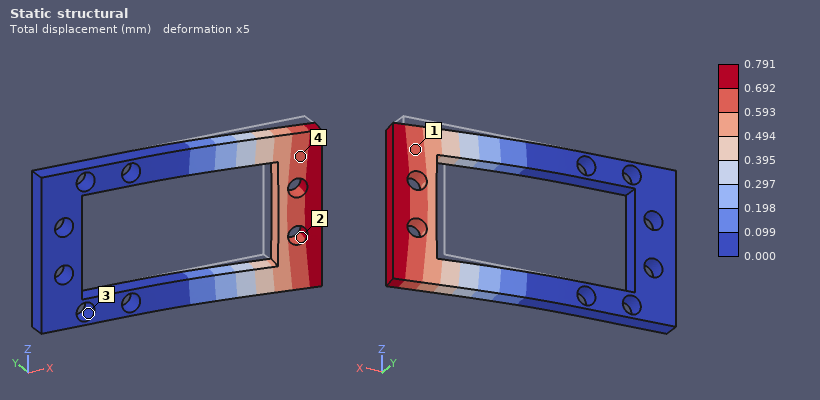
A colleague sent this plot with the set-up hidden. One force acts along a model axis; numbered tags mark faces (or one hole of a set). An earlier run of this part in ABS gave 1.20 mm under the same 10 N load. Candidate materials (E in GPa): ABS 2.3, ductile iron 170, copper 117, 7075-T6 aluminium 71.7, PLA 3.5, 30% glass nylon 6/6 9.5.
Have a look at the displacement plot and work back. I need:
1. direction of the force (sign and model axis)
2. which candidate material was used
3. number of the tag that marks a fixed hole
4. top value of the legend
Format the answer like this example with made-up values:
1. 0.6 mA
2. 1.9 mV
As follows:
1. -Y
2. PLA
3. 3
4. 0.791 mm
